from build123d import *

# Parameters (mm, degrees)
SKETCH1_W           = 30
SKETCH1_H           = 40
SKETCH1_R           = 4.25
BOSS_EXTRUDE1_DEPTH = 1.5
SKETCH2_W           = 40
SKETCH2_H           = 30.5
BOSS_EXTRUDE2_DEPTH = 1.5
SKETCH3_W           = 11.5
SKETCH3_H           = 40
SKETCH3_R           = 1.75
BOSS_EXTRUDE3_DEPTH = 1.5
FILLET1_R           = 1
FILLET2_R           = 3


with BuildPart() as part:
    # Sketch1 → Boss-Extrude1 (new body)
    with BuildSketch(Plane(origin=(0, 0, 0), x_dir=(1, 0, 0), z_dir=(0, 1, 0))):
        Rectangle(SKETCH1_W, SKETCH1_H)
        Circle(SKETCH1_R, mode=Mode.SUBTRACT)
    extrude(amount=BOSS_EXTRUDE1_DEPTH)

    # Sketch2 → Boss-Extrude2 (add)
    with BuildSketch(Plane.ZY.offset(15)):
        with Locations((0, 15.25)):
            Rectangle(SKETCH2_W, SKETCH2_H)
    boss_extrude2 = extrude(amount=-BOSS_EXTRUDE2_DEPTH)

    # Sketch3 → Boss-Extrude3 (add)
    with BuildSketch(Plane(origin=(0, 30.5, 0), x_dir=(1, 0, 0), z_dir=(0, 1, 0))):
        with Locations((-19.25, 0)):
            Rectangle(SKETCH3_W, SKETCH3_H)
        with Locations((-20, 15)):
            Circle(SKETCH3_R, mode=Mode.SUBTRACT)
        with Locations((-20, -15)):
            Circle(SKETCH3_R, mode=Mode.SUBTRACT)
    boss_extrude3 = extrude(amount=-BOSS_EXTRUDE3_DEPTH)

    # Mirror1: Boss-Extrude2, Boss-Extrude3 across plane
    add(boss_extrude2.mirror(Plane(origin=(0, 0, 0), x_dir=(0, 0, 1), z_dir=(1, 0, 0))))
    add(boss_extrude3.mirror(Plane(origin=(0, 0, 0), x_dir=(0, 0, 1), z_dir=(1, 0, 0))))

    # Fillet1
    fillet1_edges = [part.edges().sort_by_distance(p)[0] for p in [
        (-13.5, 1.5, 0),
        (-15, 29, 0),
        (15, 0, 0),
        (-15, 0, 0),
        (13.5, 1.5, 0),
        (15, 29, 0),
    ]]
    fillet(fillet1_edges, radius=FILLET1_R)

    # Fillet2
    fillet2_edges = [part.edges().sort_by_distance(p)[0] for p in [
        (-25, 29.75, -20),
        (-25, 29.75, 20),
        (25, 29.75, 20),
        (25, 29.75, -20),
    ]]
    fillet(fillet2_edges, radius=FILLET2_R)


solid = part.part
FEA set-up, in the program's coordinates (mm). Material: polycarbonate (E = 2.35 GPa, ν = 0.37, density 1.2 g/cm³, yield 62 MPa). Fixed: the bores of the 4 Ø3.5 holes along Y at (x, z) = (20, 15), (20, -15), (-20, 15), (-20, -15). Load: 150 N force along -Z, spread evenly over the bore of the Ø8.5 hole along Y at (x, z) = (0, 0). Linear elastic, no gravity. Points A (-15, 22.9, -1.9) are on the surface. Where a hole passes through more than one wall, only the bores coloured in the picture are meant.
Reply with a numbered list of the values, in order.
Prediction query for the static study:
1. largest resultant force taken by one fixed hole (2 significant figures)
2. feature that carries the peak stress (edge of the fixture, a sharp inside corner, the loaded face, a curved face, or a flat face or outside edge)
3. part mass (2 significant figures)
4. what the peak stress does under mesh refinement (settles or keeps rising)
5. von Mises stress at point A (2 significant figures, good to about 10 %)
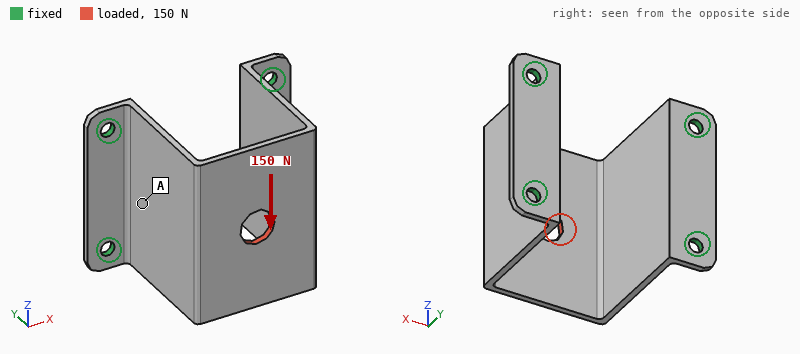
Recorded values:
1. 82 N
2. edge of the fixture
3. 7.6 g
4. keeps rising
5. 4.8 MPa
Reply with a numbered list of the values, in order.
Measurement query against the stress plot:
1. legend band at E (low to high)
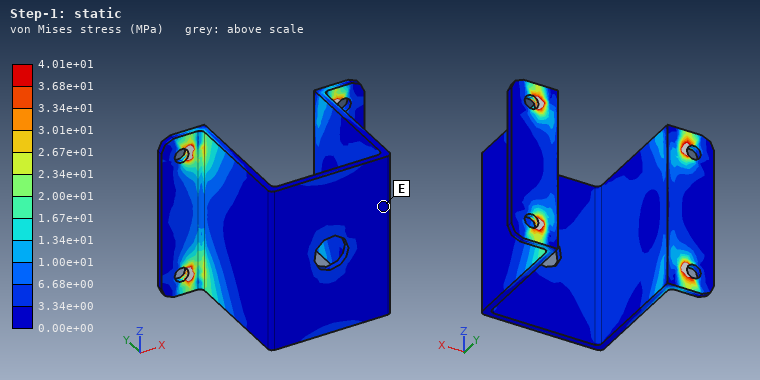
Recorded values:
1. 0.00e+00 to 3.34e+00 MPa
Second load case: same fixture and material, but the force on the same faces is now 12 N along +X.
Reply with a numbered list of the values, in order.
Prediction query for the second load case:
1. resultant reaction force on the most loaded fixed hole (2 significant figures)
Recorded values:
1. 4.5 N
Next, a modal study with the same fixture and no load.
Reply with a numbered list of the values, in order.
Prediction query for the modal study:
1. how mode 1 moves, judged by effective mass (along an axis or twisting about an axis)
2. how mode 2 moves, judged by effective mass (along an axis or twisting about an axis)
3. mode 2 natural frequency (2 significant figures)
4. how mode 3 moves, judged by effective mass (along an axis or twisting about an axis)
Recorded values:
1. along X
2. twisting about Y
3. 1100 Hz
4. along Z
